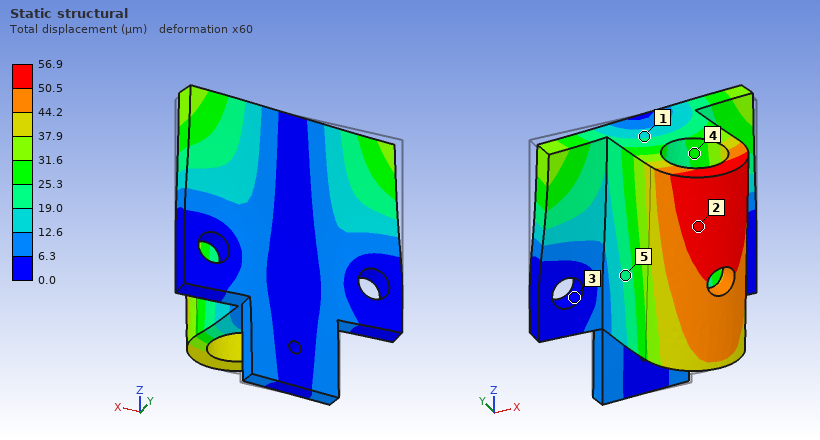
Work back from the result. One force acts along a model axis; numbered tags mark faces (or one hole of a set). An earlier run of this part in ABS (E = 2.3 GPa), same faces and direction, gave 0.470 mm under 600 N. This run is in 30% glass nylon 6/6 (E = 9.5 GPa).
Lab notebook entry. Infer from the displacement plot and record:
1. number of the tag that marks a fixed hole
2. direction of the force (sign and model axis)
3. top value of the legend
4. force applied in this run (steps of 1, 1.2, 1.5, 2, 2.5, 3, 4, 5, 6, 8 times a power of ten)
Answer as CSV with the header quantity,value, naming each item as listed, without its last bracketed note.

quantity,value
number of the tag that marks a fixed hole,3
direction of the force,+X
top value of the legend,56.9 µm
force applied in this run,300 N
